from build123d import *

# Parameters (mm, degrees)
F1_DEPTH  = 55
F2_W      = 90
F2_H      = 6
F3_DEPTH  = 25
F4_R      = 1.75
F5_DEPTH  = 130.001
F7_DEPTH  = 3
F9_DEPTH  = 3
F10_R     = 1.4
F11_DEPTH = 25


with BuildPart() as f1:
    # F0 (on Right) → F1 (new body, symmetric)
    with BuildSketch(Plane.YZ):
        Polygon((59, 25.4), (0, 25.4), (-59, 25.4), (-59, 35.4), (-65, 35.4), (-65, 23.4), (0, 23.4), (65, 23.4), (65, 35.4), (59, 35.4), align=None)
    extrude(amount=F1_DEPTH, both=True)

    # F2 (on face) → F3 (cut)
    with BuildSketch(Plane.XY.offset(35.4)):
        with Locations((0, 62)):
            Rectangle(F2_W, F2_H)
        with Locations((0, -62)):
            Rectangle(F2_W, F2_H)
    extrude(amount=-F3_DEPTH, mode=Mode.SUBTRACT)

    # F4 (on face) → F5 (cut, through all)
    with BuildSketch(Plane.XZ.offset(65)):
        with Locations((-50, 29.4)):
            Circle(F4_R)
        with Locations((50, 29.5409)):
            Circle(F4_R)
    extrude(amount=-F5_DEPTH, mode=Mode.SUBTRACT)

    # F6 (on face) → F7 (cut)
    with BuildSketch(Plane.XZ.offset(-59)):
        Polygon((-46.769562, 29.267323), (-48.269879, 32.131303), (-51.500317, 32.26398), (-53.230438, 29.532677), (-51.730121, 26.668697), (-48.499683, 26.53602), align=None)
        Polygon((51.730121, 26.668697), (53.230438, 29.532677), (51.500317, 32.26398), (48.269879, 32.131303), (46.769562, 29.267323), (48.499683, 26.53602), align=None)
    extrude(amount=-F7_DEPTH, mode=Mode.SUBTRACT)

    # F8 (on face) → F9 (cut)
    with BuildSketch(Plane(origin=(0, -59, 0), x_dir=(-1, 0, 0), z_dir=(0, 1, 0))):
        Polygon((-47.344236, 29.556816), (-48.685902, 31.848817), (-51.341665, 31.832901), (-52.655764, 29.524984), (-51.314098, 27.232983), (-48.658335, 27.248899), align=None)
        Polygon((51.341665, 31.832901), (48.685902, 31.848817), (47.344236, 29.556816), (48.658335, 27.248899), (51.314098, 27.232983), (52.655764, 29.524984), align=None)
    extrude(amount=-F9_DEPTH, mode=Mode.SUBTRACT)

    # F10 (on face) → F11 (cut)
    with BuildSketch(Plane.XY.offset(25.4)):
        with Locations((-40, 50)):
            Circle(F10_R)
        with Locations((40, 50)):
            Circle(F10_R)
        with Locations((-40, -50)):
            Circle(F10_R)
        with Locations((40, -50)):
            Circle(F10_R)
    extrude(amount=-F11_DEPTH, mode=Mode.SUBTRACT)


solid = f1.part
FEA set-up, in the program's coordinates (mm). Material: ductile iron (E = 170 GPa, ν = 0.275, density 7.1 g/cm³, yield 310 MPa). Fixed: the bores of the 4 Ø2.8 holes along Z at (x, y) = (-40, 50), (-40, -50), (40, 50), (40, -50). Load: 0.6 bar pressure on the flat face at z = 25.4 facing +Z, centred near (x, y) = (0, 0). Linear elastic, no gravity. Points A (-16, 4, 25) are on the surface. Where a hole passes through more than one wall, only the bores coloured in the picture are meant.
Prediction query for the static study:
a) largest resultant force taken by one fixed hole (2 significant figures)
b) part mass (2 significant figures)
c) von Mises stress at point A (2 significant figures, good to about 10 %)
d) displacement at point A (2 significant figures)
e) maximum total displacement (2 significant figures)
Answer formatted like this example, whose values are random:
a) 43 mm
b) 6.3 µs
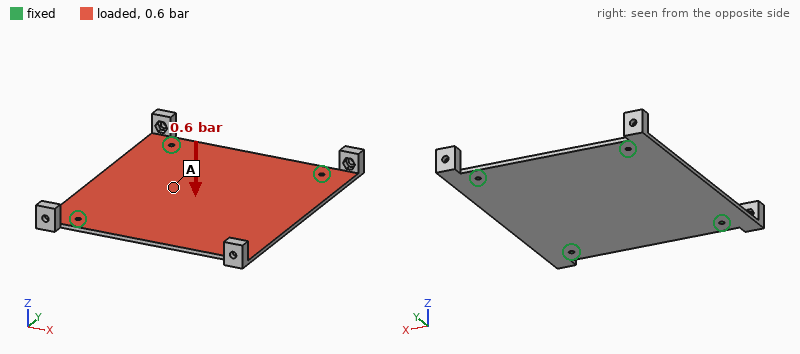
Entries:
a) 190 N
b) 200 g
c) 41 MPa
d) 0.26 mm
e) 0.27 mm
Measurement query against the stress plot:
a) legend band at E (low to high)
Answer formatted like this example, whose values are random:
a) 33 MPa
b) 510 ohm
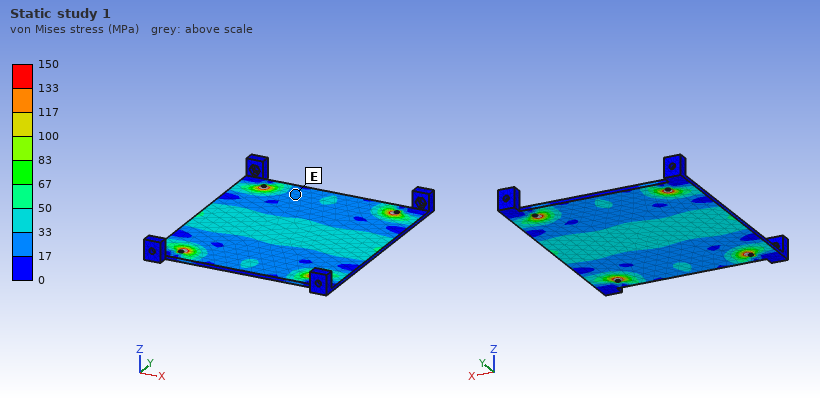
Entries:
a) 17 to 33 MPa
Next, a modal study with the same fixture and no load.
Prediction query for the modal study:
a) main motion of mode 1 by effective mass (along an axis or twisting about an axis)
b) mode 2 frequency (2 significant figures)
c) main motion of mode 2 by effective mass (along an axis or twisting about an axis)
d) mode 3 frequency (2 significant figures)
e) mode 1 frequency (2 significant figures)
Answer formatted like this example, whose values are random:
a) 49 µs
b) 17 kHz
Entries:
a) along Z
b) 1100 Hz
c) twisting about Y
d) 1400 Hz
e) 750 Hz
